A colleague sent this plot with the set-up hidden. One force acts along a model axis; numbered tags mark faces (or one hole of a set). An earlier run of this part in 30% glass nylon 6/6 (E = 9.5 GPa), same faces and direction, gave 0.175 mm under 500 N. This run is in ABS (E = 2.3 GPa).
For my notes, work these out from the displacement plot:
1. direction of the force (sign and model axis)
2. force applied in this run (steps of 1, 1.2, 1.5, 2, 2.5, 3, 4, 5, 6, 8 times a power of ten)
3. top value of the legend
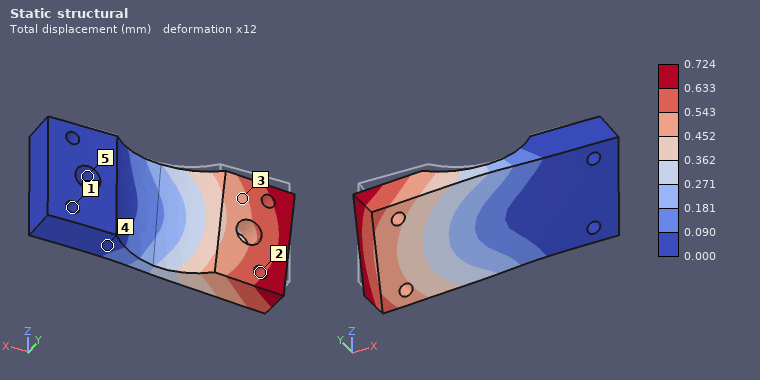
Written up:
-Z
500 N
0.724 mm
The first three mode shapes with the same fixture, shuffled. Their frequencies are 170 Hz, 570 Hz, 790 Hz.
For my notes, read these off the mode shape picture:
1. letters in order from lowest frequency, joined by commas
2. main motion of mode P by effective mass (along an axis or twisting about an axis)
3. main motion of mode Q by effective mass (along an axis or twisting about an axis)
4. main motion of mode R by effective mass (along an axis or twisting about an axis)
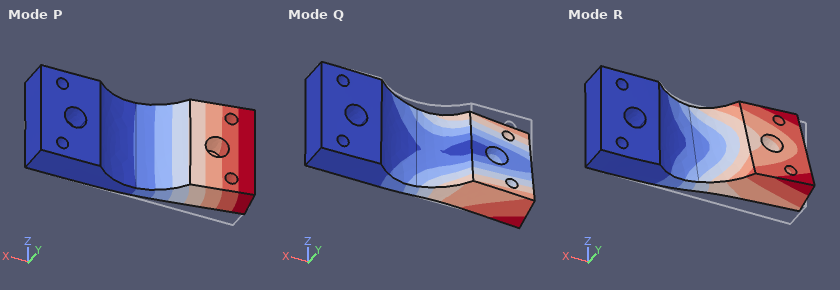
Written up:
P, R, Q
along Y
along Z
along Z
